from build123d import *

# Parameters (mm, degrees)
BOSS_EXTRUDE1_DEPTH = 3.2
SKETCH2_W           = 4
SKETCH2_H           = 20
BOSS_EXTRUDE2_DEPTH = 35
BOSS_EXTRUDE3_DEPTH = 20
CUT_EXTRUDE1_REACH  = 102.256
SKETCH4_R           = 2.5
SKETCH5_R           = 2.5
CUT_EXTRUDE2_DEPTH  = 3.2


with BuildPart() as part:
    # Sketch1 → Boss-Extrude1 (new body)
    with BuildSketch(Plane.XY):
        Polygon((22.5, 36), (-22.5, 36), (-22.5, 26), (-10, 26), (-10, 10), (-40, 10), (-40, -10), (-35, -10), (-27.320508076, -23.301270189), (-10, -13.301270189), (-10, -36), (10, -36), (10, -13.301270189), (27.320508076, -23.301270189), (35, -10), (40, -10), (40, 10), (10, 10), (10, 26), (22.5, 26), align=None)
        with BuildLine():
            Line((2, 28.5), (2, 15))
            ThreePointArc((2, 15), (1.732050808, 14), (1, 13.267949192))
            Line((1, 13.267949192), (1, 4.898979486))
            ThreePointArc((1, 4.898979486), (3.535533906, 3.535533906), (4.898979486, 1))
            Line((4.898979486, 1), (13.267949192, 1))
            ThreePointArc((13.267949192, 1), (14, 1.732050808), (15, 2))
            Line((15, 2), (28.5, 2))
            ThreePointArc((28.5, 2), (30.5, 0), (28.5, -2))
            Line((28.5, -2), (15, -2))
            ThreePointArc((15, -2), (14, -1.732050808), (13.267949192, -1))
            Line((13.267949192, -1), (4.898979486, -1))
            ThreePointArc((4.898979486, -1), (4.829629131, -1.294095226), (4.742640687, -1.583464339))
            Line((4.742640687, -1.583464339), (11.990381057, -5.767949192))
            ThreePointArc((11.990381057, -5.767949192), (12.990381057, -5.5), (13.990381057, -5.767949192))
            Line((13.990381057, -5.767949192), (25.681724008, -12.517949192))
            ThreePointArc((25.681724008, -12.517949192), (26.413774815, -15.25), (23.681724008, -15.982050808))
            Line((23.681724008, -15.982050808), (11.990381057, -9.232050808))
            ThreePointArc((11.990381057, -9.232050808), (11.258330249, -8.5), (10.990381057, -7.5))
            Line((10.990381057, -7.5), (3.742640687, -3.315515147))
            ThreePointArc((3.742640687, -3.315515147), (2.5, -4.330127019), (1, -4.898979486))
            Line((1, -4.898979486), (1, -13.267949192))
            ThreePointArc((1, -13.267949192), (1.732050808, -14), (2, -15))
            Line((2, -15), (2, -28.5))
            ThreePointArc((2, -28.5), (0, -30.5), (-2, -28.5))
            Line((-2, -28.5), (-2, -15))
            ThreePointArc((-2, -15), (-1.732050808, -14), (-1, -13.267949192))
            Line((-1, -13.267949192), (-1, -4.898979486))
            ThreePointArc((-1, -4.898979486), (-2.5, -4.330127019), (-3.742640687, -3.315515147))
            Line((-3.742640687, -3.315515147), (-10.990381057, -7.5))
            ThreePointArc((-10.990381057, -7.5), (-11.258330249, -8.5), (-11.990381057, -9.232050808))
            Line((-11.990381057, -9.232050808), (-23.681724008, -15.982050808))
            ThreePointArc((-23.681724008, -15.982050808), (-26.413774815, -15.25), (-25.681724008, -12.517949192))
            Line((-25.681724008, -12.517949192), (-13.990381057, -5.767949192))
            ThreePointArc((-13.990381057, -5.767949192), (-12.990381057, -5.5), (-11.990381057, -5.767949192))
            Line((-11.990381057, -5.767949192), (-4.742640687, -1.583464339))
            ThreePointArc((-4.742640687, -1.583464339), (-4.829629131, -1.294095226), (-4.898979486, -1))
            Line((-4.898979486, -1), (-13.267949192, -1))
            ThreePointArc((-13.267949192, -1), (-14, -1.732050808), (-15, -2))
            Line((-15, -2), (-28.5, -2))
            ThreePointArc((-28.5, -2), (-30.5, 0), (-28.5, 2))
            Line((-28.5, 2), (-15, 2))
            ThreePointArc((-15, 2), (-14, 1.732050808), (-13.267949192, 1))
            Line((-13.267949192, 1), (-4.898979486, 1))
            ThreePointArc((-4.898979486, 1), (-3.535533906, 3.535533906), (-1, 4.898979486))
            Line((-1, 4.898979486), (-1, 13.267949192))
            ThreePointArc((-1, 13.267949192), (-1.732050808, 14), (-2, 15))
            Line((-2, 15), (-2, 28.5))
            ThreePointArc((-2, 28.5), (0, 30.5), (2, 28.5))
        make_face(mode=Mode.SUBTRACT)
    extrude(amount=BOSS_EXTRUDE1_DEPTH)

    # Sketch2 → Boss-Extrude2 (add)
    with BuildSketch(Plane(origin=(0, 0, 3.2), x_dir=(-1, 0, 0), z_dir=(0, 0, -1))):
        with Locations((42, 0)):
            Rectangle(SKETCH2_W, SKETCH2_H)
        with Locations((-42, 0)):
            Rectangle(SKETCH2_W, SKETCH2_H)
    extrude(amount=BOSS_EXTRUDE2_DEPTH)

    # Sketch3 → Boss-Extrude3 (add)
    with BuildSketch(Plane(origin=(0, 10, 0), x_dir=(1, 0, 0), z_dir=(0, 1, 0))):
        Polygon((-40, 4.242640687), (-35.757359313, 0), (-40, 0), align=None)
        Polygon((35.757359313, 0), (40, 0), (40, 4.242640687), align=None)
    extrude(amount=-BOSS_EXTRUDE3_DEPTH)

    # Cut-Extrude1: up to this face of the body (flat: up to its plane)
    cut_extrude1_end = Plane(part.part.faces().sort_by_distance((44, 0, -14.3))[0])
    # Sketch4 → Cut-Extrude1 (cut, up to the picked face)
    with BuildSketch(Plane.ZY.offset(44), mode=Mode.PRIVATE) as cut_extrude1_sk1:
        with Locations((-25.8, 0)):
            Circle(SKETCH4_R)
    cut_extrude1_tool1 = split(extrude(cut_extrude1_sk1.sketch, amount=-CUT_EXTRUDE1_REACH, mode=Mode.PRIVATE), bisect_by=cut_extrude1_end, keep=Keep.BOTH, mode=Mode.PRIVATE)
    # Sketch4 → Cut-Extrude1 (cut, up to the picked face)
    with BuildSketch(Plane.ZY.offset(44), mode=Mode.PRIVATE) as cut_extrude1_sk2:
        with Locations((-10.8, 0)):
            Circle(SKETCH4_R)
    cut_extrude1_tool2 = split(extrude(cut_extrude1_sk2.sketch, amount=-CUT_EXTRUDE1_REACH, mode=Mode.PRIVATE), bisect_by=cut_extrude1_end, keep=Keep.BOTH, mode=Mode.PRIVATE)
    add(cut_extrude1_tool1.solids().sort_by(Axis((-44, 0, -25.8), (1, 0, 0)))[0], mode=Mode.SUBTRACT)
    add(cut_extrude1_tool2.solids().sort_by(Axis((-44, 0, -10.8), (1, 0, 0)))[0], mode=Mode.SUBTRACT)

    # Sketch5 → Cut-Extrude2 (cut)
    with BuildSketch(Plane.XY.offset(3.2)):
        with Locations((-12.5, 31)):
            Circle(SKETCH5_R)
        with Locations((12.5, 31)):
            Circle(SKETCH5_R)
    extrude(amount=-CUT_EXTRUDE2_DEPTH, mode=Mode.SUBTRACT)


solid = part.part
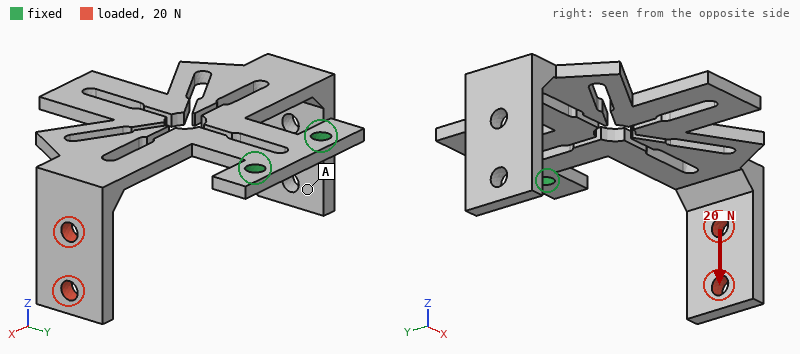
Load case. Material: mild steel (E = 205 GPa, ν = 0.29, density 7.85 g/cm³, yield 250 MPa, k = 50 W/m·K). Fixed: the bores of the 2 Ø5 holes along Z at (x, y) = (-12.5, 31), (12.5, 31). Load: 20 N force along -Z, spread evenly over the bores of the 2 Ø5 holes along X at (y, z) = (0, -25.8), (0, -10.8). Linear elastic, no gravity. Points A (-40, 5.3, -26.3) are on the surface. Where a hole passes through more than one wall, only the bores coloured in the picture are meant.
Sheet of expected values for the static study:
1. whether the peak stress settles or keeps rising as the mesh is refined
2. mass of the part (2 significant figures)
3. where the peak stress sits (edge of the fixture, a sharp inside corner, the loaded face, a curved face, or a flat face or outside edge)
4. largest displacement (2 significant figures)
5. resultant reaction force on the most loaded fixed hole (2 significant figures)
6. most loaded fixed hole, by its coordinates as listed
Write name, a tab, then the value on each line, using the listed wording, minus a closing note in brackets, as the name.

whether the peak stress settles or keeps rising as the mesh is refined	keeps rising
mass of the part	110 g
where the peak stress sits	a sharp inside corner
largest displacement	0.25 mm
resultant reaction force on the most loaded fixed hole	46 N
most loaded fixed hole, by its coordinates as listed	(12.5, 31)
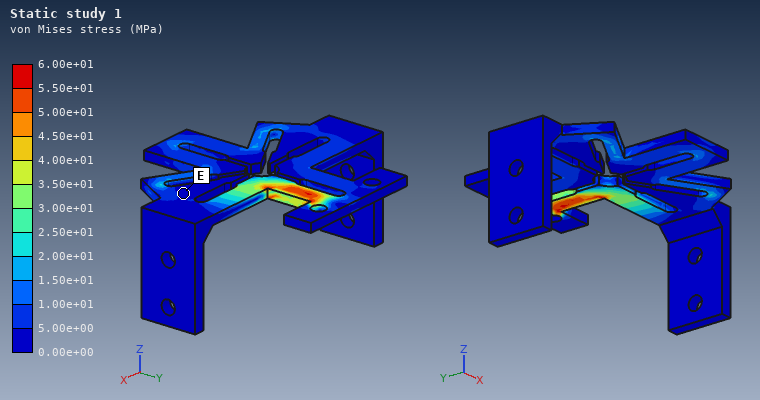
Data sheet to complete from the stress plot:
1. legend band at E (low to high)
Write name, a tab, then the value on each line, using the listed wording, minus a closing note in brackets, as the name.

legend band at E	0.00e+00 to 5.00e+00 MPa
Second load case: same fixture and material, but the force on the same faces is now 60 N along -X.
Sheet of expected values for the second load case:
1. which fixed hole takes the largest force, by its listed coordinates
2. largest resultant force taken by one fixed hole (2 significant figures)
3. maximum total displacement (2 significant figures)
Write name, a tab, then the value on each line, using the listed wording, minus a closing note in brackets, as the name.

which fixed hole takes the largest force, by its listed coordinates	(12.5, 31)
largest resultant force taken by one fixed hole	100 N
maximum total displacement	0.43 mm
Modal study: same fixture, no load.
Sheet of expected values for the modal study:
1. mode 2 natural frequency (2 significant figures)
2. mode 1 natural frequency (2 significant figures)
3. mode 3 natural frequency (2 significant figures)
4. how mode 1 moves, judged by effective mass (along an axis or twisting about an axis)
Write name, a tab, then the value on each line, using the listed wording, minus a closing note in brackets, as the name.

mode 2 natural frequency	280 Hz
mode 1 natural frequency	270 Hz
mode 3 natural frequency	460 Hz
how mode 1 moves, judged by effective mass	along Z
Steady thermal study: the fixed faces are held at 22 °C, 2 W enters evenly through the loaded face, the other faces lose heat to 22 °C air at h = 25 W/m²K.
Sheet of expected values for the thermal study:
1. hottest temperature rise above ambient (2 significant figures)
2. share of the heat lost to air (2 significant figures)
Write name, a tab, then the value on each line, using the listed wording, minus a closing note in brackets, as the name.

hottest temperature rise above ambient	24 K
share of the heat lost to air	83 %
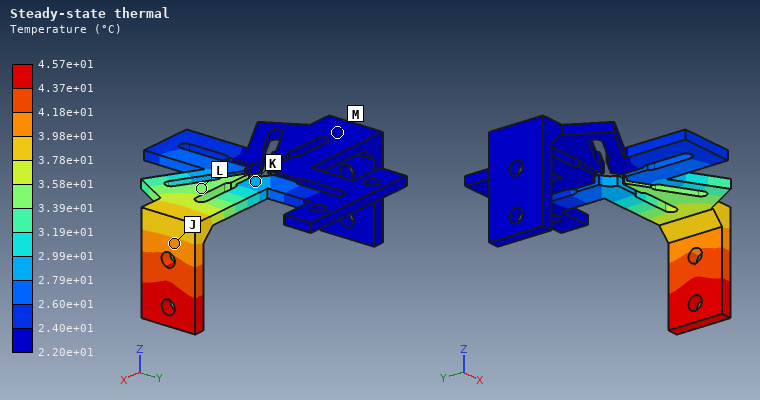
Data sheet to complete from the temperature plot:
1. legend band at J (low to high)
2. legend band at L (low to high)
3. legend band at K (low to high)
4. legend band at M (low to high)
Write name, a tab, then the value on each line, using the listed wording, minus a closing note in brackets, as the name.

legend band at J	3.98e+01 to 4.18e+01 °C
legend band at L	3.39e+01 to 3.58e+01 °C
legend band at K	2.79e+01 to 2.99e+01 °C
legend band at M	2.20e+01 to 2.40e+01 °C
